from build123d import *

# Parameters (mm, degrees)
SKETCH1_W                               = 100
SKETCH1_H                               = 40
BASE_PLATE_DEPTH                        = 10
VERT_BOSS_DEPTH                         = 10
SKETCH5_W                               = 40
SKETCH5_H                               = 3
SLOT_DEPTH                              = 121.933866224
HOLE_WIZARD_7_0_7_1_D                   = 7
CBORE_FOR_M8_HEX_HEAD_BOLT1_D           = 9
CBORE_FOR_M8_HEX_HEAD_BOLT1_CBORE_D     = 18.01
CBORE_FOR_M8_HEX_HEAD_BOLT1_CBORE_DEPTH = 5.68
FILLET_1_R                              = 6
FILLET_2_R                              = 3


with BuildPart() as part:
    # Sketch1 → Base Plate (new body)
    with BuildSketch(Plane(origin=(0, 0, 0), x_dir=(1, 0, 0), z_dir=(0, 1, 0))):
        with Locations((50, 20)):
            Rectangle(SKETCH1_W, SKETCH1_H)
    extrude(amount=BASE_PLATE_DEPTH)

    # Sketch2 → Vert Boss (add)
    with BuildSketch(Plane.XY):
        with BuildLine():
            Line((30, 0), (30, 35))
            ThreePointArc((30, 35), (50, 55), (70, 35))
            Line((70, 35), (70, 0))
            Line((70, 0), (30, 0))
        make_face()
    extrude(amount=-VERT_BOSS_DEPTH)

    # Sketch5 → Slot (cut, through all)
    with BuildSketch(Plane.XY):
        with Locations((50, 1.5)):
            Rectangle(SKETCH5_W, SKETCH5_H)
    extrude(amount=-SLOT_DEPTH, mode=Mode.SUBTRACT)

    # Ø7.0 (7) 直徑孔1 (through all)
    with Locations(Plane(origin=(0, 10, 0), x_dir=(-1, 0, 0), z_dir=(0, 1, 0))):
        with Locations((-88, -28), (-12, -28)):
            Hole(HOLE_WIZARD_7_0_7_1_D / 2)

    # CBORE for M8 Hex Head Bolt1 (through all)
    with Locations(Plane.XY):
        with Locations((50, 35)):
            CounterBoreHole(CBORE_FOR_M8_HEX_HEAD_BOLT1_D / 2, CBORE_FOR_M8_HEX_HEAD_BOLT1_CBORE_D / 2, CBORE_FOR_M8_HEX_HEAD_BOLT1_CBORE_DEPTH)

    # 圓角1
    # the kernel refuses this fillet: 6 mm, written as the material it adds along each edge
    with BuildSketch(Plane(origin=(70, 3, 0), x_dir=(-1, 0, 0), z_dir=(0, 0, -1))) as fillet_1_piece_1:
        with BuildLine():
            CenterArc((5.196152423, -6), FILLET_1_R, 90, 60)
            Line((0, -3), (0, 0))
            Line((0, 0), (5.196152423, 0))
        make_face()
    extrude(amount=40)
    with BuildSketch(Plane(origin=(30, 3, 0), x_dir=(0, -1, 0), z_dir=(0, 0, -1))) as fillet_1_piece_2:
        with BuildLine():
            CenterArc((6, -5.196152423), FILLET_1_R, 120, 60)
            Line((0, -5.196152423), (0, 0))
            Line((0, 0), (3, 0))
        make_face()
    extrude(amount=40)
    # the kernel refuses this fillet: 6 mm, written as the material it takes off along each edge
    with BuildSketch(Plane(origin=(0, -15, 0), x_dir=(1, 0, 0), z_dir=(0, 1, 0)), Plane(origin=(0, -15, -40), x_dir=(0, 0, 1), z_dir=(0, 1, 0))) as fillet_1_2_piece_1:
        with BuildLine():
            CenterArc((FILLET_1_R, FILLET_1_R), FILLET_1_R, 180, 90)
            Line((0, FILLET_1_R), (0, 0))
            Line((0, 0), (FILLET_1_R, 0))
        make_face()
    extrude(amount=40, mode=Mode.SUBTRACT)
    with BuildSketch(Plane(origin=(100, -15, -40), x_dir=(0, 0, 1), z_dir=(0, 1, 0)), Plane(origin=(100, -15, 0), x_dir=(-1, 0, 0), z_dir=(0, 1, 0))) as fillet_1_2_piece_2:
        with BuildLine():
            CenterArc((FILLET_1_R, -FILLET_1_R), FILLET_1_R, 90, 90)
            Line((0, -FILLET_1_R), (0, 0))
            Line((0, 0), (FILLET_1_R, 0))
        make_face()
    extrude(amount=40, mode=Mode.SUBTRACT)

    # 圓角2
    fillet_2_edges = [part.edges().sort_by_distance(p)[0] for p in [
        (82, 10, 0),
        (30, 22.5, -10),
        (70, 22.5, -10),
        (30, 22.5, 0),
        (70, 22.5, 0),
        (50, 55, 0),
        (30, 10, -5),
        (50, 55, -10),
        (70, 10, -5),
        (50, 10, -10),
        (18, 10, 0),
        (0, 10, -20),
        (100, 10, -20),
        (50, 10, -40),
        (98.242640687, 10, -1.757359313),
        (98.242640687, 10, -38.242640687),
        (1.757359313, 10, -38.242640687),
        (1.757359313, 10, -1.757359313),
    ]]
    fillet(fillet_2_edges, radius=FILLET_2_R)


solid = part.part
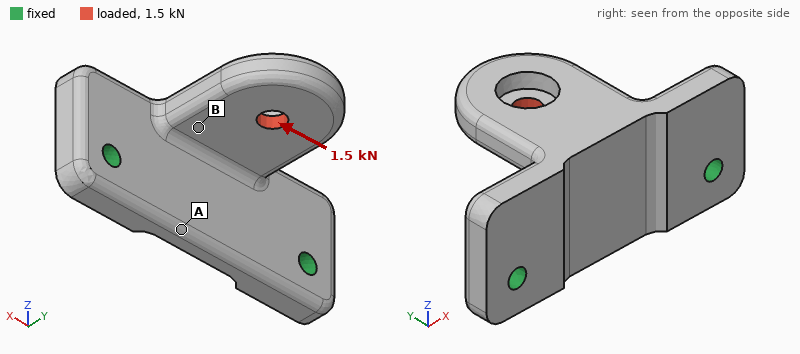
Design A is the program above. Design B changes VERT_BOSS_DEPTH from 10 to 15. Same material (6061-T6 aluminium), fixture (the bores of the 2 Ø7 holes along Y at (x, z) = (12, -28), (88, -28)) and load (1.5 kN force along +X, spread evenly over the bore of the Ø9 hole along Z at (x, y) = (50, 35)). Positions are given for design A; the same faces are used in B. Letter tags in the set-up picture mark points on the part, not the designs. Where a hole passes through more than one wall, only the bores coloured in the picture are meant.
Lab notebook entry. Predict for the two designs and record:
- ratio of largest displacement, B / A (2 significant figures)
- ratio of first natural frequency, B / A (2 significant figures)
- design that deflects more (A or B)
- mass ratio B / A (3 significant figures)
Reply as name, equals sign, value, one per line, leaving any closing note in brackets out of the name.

ratio of largest displacement, B / A = 0.66
ratio of first natural frequency, B / A = 0.96
design that deflects more = A
mass ratio B / A = 1.16
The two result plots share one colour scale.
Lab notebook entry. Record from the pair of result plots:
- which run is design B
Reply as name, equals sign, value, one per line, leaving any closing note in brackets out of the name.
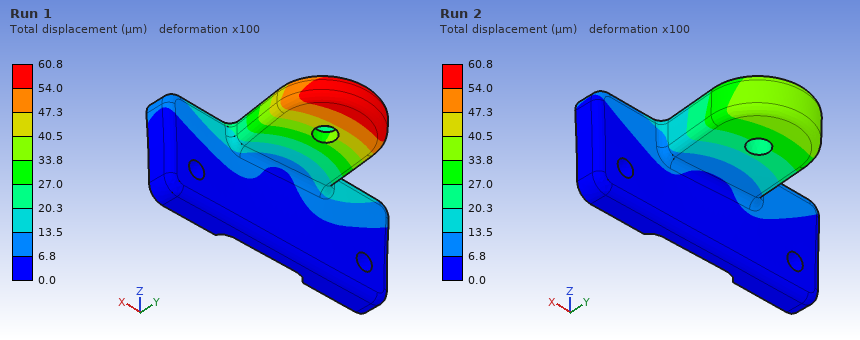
which run is design B = Run 2
